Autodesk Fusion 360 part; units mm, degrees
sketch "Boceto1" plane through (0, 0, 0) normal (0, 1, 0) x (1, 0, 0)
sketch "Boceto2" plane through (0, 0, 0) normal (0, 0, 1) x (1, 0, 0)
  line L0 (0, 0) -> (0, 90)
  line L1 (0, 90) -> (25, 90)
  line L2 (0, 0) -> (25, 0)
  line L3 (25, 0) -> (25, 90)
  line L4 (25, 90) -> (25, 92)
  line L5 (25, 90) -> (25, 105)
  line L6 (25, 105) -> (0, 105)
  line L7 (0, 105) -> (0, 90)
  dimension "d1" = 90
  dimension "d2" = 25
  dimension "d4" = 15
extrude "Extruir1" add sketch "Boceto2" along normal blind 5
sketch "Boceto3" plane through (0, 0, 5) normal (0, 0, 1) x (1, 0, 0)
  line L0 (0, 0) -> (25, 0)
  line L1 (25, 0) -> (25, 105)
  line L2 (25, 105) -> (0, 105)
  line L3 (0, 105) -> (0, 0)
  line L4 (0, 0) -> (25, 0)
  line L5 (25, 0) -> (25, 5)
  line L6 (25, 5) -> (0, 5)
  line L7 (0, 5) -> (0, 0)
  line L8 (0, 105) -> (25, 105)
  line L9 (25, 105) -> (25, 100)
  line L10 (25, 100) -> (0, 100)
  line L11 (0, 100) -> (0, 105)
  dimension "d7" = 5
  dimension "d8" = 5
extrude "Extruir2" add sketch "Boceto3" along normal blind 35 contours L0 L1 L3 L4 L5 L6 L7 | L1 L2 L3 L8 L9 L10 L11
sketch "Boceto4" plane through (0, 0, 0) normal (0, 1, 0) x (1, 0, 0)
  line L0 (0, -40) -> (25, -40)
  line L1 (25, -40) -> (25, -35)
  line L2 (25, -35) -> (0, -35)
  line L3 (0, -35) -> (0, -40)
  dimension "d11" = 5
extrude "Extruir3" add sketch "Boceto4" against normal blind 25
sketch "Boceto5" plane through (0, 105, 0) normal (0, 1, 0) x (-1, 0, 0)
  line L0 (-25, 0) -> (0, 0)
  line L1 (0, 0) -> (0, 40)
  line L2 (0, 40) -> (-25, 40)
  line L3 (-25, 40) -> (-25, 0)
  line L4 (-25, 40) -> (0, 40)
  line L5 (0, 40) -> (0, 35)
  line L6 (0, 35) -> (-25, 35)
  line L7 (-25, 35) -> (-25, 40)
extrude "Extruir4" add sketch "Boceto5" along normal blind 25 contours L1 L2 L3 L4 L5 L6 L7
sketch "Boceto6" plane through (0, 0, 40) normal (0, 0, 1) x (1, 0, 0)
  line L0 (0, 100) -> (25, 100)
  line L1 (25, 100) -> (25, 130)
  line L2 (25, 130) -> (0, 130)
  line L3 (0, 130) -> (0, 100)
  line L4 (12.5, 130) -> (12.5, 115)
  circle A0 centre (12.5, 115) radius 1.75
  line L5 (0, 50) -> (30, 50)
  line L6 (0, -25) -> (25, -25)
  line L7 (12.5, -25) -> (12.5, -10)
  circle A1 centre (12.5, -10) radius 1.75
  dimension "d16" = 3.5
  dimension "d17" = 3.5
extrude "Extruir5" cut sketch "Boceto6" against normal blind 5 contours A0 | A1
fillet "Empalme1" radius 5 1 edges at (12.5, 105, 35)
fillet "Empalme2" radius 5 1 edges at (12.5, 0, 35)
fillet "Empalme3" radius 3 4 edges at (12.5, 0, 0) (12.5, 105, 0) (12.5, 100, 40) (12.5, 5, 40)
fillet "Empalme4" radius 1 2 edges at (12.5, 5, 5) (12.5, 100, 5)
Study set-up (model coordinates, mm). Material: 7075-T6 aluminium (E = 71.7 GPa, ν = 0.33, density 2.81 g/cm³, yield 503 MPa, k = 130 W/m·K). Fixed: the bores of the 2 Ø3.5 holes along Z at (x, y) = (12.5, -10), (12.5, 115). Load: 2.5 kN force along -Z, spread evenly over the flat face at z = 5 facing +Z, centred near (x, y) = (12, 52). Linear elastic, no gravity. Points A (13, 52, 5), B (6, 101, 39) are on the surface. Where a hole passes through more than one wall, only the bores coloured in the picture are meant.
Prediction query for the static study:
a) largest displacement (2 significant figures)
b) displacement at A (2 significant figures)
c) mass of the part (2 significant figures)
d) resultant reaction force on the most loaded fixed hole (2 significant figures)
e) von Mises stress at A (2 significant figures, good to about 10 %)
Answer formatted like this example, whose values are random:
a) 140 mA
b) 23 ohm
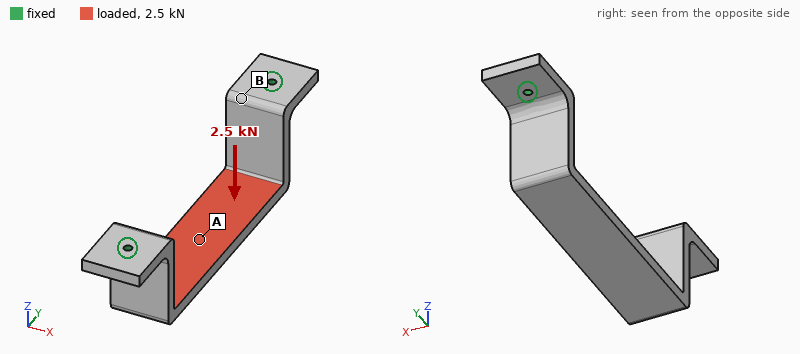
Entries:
a) 0.55 mm
b) 0.54 mm
c) 79 g
d) 1.5 kN
e) 120 MPa
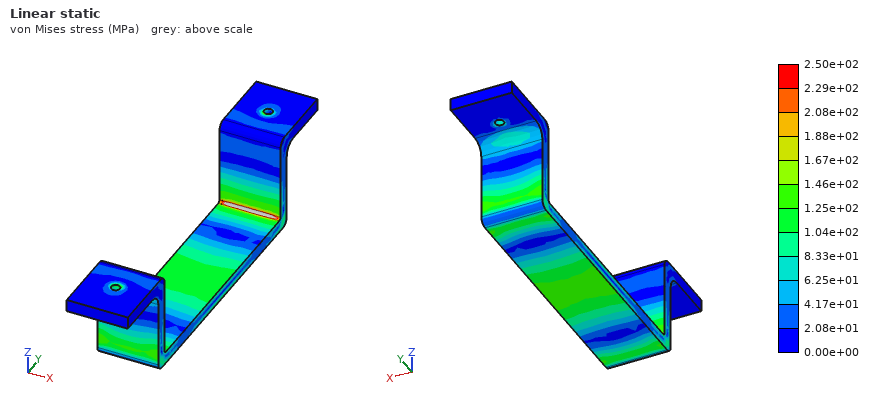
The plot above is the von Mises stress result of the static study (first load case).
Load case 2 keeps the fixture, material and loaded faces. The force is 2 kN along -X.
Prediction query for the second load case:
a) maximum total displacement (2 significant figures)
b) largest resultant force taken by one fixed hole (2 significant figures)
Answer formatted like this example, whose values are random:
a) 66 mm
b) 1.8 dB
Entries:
a) 0.59 mm
b) 1.0 kN
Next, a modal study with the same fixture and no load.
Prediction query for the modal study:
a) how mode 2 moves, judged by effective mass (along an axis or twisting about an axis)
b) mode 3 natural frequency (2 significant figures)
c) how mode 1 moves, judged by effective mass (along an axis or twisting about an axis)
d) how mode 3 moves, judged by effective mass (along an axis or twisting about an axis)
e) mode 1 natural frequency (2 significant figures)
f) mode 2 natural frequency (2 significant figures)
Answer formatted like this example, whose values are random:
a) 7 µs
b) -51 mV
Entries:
a) along Y
b) 2100 Hz
c) along X
d) along Z
e) 1400 Hz
f) 1500 Hz
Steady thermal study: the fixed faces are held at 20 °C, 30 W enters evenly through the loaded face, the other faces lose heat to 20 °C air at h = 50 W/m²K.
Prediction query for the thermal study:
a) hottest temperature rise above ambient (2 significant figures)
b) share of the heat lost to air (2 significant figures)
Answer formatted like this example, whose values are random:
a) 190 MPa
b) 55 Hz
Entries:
a) 46 K
b) 37 %
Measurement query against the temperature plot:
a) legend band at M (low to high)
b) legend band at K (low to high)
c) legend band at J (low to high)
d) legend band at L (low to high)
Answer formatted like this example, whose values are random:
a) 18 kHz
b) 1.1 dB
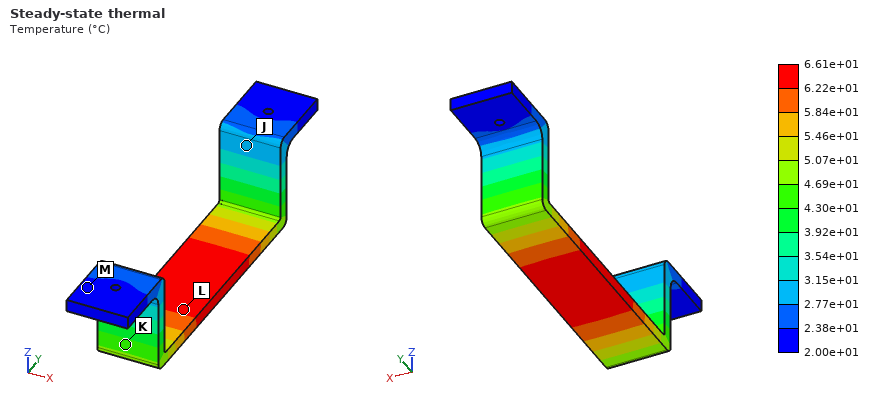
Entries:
a) 2.00e+01 to 2.38e+01 °C
b) 4.30e+01 to 4.69e+01 °C
c) 2.77e+01 to 3.15e+01 °C
d) 6.22e+01 to 6.61e+01 °C
